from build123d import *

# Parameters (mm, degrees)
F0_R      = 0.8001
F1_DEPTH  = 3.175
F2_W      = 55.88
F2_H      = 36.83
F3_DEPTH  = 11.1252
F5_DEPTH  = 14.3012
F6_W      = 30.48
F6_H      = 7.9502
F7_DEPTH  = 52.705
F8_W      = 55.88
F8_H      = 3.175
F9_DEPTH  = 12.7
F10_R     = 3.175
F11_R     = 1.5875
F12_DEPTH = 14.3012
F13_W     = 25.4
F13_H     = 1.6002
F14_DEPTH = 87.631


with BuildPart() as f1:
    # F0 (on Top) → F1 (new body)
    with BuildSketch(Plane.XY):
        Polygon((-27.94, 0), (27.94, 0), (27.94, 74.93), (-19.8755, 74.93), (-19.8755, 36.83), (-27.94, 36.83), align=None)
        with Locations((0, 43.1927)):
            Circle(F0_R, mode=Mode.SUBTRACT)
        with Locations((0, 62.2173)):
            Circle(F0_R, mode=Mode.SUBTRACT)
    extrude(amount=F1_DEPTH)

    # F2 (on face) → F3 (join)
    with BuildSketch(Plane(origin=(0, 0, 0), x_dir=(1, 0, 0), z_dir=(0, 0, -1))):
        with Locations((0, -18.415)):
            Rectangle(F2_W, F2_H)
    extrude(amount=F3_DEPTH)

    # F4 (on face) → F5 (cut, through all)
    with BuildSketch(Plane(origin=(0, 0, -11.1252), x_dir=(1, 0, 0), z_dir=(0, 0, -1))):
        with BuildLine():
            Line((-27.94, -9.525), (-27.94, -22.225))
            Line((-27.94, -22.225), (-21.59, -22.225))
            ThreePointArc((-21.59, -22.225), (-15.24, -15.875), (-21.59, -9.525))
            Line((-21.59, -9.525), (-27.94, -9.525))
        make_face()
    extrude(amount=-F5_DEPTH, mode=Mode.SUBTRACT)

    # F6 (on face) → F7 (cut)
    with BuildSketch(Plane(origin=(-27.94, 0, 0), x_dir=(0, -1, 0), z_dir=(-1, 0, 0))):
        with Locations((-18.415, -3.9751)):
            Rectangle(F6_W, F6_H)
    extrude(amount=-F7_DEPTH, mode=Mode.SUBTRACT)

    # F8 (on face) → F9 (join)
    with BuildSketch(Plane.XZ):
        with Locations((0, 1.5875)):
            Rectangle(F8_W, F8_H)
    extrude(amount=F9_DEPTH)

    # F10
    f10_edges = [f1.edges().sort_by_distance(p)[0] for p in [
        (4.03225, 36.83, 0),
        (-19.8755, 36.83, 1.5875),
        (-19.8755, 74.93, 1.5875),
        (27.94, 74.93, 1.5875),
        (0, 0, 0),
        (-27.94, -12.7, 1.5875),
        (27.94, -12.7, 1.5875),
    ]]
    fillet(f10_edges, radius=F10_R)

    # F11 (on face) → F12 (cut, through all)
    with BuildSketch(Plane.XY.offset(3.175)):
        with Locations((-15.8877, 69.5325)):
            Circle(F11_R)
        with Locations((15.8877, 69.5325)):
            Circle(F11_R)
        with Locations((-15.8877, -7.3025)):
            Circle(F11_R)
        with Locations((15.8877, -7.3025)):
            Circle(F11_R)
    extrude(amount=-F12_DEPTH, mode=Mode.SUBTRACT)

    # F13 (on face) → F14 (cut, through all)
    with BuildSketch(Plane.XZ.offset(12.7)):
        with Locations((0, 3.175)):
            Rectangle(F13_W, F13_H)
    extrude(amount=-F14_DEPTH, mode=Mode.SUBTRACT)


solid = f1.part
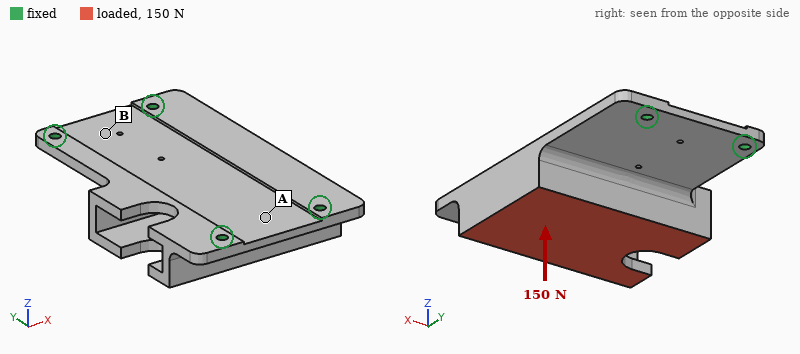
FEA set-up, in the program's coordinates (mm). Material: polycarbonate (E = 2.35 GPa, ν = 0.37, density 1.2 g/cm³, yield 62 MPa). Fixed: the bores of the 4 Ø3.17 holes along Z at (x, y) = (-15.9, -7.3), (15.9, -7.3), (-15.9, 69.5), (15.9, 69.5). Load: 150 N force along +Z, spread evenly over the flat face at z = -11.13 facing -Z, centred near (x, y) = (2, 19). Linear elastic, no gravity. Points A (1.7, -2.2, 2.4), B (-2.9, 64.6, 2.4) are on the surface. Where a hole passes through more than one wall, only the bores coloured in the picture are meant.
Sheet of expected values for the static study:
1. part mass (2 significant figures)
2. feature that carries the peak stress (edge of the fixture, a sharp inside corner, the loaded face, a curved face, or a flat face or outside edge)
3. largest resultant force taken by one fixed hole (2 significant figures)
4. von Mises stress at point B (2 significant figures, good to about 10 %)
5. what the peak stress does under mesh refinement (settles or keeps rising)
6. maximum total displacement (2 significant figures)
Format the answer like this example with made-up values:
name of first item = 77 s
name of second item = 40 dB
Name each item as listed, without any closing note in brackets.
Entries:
part mass = 27 g
feature that carries the peak stress = edge of the fixture
largest resultant force taken by one fixed hole = 57 N
von Mises stress at point B = 4.0 MPa
what the peak stress does under mesh refinement = keeps rising
maximum total displacement = 0.66 mm
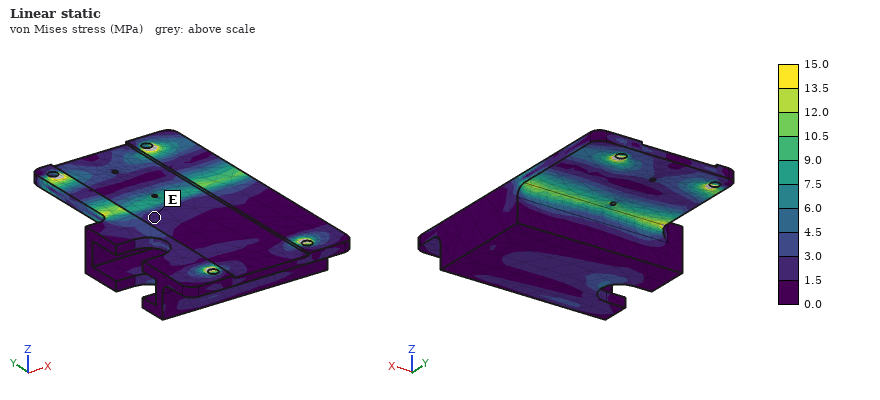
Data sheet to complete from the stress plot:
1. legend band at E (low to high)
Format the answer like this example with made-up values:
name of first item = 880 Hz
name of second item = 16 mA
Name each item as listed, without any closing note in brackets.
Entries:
legend band at E = 1.5 to 3.0 MPa
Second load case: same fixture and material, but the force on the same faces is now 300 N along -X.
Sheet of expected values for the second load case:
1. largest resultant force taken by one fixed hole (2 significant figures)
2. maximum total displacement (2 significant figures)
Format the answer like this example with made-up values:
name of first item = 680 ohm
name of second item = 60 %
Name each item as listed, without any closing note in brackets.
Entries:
largest resultant force taken by one fixed hole = 190 N
maximum total displacement = 0.40 mm
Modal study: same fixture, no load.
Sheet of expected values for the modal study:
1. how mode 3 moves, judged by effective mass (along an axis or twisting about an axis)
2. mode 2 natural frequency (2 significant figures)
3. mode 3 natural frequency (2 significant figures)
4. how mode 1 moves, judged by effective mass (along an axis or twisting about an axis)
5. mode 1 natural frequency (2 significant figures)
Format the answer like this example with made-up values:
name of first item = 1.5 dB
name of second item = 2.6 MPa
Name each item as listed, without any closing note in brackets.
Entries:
how mode 3 moves, judged by effective mass = along Y
mode 2 natural frequency = 1200 Hz
mode 3 natural frequency = 2300 Hz
how mode 1 moves, judged by effective mass = along Z
mode 1 natural frequency = 590 Hz
